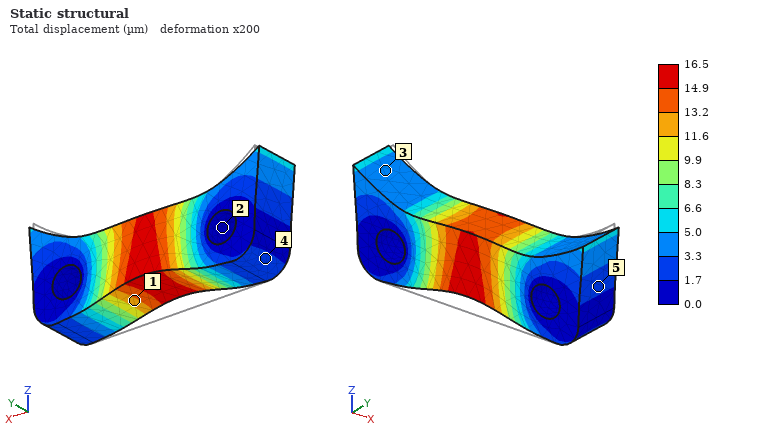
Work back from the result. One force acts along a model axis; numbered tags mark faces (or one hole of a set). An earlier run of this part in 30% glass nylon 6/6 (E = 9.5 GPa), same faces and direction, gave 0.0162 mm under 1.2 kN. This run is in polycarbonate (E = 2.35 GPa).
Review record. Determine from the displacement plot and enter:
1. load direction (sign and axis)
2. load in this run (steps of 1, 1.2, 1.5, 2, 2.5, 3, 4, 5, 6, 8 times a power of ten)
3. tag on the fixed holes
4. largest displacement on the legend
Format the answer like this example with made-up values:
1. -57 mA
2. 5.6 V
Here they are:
1. +Z
2. 300 N
3. 2
4. 16.5 µm
